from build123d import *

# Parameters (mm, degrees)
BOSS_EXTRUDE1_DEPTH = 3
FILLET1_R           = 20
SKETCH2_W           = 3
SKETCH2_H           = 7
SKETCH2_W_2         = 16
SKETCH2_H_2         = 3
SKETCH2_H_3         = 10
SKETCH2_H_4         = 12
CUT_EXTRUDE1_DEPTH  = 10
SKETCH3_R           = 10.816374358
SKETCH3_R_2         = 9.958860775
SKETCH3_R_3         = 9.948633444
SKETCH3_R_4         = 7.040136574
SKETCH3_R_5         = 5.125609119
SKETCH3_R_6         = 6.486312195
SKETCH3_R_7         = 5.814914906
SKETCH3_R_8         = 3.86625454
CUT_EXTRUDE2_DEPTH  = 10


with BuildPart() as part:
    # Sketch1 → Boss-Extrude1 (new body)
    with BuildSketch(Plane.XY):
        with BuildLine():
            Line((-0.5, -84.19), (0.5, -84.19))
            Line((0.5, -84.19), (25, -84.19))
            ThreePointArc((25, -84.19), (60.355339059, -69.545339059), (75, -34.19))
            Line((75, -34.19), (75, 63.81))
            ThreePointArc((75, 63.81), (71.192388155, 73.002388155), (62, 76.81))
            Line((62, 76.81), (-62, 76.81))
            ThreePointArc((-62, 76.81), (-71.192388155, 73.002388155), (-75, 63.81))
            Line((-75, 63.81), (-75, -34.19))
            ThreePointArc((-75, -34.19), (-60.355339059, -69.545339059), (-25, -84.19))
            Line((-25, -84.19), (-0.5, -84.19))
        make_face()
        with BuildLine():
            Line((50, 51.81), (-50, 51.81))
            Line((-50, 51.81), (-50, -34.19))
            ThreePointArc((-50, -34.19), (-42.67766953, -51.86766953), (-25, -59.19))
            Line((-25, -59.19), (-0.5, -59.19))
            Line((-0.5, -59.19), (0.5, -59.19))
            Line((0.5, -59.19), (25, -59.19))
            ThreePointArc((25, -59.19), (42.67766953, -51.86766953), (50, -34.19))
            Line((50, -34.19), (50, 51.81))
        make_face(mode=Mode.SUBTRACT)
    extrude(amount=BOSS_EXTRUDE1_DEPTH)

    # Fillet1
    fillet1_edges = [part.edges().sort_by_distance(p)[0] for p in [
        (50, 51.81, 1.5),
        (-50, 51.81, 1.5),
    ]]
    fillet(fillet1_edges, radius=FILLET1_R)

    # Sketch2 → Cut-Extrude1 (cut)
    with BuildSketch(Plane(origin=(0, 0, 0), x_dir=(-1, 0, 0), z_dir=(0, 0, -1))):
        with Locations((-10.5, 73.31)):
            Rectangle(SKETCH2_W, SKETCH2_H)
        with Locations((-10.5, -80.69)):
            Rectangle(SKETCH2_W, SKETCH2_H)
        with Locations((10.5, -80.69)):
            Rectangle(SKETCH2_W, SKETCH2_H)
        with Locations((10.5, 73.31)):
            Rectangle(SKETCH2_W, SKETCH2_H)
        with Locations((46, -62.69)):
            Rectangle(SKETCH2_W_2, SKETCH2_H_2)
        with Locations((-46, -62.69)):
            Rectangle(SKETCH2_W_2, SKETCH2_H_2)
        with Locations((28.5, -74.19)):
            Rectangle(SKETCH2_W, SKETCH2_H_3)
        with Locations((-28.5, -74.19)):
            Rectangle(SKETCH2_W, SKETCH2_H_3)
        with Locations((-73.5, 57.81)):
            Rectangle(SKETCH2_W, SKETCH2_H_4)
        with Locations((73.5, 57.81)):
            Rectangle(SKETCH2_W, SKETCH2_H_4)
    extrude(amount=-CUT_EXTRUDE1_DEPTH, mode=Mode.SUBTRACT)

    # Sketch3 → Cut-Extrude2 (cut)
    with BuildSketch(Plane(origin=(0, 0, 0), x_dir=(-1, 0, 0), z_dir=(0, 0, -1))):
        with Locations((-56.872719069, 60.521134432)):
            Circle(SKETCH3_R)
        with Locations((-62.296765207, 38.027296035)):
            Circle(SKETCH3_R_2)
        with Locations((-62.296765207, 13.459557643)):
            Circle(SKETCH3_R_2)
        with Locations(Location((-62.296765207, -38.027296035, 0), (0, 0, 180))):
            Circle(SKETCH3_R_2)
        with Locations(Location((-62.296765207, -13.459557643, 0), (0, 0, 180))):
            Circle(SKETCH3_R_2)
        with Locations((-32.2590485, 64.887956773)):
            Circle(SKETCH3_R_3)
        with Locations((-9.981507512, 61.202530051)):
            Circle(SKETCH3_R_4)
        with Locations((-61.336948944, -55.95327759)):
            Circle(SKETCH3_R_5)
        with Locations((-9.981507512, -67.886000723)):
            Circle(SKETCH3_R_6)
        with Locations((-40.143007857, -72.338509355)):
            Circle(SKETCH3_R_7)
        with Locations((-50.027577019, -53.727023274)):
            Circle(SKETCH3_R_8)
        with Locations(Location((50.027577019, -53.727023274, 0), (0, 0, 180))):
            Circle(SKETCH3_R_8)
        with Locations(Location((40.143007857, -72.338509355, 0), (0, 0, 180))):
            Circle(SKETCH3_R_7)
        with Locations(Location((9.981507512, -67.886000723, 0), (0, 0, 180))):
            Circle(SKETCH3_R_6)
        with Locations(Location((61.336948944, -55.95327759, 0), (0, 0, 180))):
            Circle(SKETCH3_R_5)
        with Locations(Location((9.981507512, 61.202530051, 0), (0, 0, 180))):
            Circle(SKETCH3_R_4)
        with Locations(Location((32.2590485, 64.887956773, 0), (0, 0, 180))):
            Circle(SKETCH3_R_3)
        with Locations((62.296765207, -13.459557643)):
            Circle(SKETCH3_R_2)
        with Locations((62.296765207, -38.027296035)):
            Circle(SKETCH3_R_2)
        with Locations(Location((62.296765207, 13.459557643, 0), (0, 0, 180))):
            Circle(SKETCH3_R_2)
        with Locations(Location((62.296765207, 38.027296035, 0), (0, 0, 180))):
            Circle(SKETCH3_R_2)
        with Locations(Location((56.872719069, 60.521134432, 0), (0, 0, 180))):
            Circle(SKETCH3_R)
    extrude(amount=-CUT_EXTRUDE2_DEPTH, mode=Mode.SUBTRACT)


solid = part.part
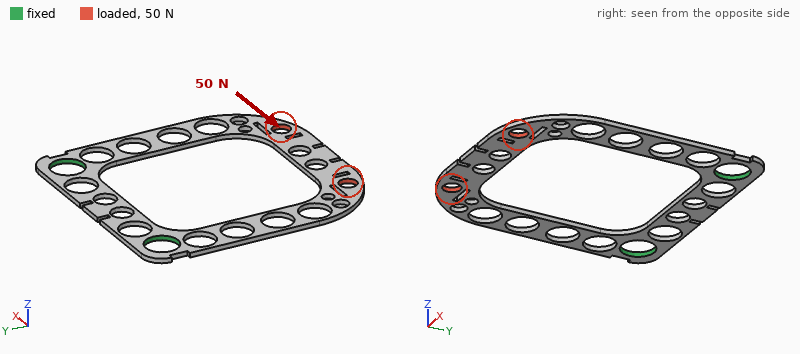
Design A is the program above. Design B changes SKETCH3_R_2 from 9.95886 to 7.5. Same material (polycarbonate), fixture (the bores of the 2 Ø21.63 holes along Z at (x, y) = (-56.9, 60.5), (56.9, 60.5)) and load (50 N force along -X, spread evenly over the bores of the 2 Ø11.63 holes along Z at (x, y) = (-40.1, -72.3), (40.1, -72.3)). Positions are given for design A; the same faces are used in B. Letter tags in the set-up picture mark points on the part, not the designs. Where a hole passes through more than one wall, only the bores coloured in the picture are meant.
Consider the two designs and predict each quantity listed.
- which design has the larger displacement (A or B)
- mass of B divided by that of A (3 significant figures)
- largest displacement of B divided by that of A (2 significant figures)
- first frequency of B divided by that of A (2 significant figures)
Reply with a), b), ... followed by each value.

a) A
b) 1.15
c) 0.56
d) 1.3
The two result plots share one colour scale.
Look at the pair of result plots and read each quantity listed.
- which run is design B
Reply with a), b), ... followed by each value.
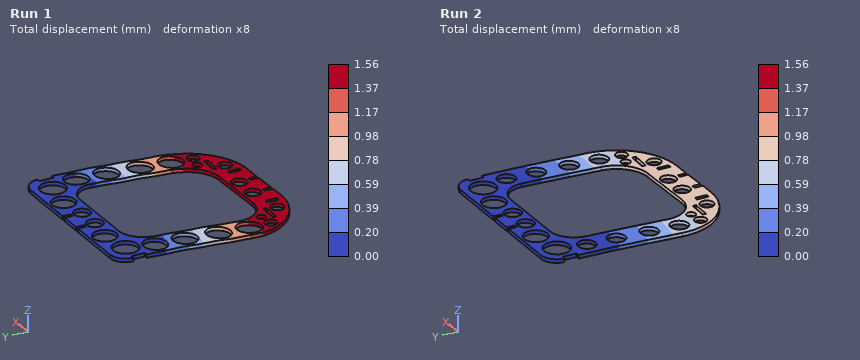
a) Run 2
